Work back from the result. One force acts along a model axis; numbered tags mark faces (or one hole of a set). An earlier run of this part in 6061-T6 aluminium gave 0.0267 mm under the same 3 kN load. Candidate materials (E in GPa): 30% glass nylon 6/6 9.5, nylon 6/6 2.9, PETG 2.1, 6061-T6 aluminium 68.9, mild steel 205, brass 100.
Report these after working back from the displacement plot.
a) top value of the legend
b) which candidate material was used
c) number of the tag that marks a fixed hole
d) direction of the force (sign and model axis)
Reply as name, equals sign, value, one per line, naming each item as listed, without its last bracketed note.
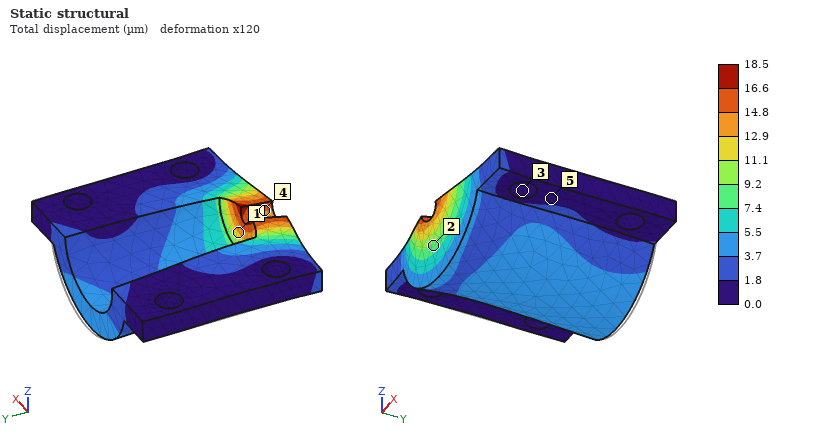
top value of the legend = 18.5 µm
which candidate material was used = brass
number of the tag that marks a fixed hole = 3
direction of the force = -Y
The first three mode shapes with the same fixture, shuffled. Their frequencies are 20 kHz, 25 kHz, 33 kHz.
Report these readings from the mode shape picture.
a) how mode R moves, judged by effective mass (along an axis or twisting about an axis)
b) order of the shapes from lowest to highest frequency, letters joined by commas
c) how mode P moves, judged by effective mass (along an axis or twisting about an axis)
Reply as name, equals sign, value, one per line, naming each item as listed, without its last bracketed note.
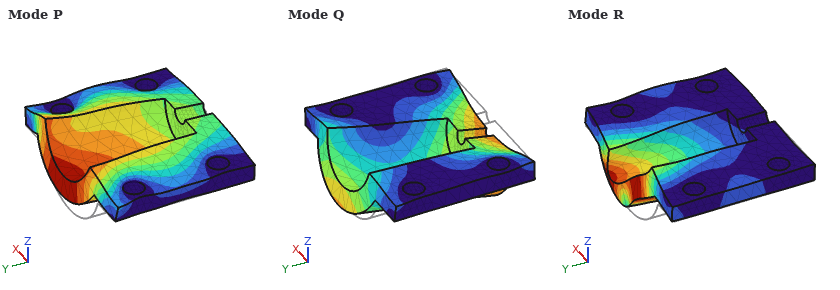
how mode R moves, judged by effective mass = along X
order of the shapes from lowest to highest frequency, letters joined by commas = Q, P, R
how mode P moves, judged by effective mass = along Z
